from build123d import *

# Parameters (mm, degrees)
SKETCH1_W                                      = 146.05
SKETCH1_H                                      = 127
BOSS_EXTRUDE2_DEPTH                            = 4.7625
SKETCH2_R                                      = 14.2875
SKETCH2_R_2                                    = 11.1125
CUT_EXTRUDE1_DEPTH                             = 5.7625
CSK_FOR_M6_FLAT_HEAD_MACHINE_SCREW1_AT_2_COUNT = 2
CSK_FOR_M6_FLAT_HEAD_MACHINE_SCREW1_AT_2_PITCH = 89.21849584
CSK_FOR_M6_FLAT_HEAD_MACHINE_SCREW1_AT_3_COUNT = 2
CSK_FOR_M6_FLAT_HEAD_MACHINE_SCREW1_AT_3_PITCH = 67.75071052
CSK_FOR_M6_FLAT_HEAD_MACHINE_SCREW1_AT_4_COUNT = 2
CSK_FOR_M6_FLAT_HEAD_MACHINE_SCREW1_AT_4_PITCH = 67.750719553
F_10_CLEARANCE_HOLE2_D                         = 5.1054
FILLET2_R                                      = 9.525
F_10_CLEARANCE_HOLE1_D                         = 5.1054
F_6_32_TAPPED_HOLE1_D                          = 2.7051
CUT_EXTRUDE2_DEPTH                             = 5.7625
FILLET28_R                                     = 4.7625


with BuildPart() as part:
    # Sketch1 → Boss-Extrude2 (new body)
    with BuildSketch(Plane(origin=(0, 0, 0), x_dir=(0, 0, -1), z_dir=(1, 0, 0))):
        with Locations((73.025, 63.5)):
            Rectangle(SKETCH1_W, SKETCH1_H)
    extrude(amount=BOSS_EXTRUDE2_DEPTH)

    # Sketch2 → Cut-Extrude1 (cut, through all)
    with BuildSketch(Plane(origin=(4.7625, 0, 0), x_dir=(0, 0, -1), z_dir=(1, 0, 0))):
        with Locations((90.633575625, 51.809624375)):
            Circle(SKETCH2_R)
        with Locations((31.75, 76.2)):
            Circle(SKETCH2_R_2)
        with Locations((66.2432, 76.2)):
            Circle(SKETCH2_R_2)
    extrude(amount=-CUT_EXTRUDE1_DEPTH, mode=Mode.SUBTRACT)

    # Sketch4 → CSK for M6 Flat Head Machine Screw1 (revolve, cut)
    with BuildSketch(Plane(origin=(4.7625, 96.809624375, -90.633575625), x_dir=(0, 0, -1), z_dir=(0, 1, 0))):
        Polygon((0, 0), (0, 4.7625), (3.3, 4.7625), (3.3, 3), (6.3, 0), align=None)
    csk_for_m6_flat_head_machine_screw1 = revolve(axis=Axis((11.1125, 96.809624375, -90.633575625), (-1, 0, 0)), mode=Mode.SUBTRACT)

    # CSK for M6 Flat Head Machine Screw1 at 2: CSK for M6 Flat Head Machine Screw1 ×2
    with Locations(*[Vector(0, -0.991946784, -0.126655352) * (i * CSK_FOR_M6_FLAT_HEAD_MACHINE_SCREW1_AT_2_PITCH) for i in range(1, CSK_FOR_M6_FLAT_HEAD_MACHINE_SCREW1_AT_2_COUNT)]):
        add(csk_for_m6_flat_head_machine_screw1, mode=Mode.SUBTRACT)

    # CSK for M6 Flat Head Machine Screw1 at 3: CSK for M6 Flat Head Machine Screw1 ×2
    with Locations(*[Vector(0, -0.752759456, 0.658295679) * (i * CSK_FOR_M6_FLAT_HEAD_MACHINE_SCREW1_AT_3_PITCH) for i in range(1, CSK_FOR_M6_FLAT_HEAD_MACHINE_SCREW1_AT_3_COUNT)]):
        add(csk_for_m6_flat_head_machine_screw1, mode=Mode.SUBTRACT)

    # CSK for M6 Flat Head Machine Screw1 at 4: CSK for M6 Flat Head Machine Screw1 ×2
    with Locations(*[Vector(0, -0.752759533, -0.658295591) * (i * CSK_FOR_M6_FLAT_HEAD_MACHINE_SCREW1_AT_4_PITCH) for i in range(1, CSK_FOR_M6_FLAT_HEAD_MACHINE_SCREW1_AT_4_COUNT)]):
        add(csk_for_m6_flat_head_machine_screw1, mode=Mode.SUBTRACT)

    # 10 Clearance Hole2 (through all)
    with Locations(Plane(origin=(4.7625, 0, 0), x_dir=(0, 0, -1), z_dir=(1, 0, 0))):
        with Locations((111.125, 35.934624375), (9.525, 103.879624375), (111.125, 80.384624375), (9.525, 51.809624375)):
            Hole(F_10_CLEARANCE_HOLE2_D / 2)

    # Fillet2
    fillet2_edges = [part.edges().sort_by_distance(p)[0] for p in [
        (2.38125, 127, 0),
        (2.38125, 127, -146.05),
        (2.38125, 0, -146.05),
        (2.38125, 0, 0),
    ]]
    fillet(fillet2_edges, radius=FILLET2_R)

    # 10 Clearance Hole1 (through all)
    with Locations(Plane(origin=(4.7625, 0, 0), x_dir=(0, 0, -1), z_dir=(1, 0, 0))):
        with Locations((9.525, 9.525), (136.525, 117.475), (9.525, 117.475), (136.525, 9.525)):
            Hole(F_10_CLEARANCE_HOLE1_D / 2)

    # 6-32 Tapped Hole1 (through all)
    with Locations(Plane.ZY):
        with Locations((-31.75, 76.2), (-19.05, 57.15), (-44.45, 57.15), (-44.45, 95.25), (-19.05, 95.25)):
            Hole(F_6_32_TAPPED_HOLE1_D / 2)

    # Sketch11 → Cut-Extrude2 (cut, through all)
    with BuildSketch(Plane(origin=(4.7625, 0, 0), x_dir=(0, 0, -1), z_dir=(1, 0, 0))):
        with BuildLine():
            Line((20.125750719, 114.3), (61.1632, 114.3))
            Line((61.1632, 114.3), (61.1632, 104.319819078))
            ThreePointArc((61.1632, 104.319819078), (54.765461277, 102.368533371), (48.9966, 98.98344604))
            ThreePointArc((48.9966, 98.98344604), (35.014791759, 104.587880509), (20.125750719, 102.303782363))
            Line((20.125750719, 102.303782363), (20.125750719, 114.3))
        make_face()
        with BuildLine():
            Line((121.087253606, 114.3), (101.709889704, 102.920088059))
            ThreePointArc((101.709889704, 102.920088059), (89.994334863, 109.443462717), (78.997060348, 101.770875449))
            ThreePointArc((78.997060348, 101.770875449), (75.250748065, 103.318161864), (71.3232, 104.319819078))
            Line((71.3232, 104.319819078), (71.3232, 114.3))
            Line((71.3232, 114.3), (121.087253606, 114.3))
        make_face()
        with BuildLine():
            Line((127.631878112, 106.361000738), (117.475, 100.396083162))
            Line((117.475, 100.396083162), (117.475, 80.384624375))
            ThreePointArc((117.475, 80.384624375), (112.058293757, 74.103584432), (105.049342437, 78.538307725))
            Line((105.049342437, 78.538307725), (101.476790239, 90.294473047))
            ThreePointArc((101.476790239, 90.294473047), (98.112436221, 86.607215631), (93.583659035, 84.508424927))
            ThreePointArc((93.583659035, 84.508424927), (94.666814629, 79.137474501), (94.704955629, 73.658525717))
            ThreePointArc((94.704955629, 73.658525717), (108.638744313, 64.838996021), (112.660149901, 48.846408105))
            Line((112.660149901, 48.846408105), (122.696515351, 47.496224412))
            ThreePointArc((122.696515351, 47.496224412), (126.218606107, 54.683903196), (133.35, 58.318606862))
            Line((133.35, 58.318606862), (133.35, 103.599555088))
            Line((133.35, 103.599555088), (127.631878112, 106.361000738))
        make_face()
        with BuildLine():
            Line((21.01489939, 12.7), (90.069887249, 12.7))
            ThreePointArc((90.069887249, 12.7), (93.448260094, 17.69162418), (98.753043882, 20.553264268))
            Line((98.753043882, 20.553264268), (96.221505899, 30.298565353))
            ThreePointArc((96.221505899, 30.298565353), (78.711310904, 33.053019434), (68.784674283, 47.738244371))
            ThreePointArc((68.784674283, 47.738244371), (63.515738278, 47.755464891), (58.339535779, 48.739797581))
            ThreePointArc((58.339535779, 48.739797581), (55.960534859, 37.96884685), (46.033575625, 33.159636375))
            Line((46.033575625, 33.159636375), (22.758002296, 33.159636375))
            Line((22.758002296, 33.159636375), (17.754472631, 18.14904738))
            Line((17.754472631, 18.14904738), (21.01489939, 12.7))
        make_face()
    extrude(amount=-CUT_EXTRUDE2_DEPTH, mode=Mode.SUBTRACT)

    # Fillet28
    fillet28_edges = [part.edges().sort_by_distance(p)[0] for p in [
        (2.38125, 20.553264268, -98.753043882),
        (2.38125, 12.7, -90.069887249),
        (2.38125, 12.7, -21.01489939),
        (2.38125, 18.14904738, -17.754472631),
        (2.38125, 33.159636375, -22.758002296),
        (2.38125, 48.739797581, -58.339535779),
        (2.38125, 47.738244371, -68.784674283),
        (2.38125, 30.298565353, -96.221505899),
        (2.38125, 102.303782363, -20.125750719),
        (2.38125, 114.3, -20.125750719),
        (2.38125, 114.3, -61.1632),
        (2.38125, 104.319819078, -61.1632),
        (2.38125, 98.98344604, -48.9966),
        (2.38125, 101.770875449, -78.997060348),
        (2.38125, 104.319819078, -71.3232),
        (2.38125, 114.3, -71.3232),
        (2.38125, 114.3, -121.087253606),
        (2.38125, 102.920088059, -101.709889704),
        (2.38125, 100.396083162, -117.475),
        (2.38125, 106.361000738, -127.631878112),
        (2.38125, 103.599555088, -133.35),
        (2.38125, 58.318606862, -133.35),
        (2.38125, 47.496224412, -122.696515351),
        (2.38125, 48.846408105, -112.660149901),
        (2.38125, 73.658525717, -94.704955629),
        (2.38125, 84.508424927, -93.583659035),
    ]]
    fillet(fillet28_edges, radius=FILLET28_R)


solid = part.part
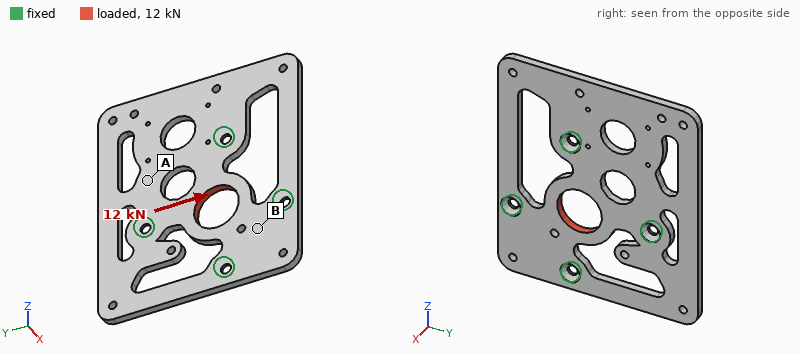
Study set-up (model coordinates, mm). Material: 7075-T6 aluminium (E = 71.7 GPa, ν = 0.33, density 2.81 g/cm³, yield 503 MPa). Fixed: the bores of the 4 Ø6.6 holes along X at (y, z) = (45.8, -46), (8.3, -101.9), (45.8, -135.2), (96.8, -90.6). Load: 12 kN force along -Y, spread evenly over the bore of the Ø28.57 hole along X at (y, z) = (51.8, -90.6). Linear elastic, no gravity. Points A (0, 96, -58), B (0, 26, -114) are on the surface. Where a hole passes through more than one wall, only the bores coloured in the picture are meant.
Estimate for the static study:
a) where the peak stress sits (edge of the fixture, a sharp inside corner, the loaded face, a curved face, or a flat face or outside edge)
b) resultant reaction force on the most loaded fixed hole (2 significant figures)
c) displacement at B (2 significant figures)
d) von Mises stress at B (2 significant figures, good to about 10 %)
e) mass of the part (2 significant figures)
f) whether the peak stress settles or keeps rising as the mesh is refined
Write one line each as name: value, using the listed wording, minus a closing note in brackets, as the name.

where the peak stress sits: edge of the fixture
resultant reaction force on the most loaded fixed hole: 4.1 kN
displacement at B: 12 µm
von Mises stress at B: 19 MPa
mass of the part: 170 g
whether the peak stress settles or keeps rising as the mesh is refined: keeps rising
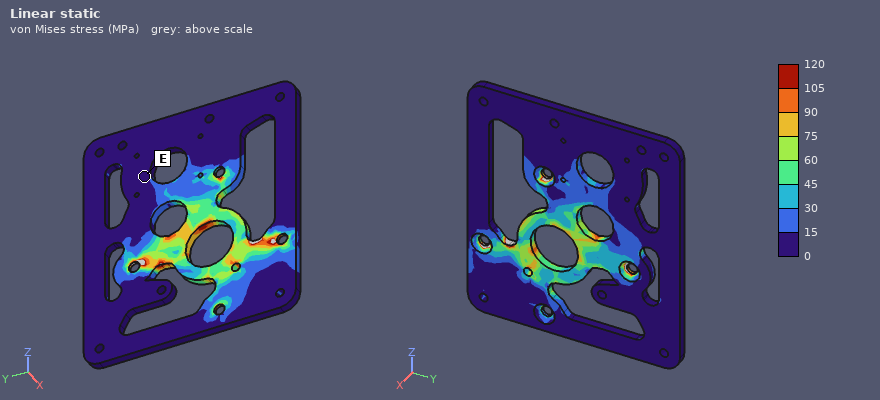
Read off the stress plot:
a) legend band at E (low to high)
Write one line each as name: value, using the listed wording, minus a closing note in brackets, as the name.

legend band at E: 0 to 15 MPa
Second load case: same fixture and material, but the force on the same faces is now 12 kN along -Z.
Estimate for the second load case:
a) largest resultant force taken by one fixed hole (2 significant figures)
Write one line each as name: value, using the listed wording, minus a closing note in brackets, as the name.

largest resultant force taken by one fixed hole: 4.0 kN
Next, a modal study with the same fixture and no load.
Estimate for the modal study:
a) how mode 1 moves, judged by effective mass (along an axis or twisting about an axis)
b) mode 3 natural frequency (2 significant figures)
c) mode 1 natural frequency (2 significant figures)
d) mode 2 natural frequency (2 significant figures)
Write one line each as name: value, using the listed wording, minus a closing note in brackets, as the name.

how mode 1 moves, judged by effective mass: along X
mode 3 natural frequency: 1100 Hz
mode 1 natural frequency: 670 Hz
mode 2 natural frequency: 1000 Hz
